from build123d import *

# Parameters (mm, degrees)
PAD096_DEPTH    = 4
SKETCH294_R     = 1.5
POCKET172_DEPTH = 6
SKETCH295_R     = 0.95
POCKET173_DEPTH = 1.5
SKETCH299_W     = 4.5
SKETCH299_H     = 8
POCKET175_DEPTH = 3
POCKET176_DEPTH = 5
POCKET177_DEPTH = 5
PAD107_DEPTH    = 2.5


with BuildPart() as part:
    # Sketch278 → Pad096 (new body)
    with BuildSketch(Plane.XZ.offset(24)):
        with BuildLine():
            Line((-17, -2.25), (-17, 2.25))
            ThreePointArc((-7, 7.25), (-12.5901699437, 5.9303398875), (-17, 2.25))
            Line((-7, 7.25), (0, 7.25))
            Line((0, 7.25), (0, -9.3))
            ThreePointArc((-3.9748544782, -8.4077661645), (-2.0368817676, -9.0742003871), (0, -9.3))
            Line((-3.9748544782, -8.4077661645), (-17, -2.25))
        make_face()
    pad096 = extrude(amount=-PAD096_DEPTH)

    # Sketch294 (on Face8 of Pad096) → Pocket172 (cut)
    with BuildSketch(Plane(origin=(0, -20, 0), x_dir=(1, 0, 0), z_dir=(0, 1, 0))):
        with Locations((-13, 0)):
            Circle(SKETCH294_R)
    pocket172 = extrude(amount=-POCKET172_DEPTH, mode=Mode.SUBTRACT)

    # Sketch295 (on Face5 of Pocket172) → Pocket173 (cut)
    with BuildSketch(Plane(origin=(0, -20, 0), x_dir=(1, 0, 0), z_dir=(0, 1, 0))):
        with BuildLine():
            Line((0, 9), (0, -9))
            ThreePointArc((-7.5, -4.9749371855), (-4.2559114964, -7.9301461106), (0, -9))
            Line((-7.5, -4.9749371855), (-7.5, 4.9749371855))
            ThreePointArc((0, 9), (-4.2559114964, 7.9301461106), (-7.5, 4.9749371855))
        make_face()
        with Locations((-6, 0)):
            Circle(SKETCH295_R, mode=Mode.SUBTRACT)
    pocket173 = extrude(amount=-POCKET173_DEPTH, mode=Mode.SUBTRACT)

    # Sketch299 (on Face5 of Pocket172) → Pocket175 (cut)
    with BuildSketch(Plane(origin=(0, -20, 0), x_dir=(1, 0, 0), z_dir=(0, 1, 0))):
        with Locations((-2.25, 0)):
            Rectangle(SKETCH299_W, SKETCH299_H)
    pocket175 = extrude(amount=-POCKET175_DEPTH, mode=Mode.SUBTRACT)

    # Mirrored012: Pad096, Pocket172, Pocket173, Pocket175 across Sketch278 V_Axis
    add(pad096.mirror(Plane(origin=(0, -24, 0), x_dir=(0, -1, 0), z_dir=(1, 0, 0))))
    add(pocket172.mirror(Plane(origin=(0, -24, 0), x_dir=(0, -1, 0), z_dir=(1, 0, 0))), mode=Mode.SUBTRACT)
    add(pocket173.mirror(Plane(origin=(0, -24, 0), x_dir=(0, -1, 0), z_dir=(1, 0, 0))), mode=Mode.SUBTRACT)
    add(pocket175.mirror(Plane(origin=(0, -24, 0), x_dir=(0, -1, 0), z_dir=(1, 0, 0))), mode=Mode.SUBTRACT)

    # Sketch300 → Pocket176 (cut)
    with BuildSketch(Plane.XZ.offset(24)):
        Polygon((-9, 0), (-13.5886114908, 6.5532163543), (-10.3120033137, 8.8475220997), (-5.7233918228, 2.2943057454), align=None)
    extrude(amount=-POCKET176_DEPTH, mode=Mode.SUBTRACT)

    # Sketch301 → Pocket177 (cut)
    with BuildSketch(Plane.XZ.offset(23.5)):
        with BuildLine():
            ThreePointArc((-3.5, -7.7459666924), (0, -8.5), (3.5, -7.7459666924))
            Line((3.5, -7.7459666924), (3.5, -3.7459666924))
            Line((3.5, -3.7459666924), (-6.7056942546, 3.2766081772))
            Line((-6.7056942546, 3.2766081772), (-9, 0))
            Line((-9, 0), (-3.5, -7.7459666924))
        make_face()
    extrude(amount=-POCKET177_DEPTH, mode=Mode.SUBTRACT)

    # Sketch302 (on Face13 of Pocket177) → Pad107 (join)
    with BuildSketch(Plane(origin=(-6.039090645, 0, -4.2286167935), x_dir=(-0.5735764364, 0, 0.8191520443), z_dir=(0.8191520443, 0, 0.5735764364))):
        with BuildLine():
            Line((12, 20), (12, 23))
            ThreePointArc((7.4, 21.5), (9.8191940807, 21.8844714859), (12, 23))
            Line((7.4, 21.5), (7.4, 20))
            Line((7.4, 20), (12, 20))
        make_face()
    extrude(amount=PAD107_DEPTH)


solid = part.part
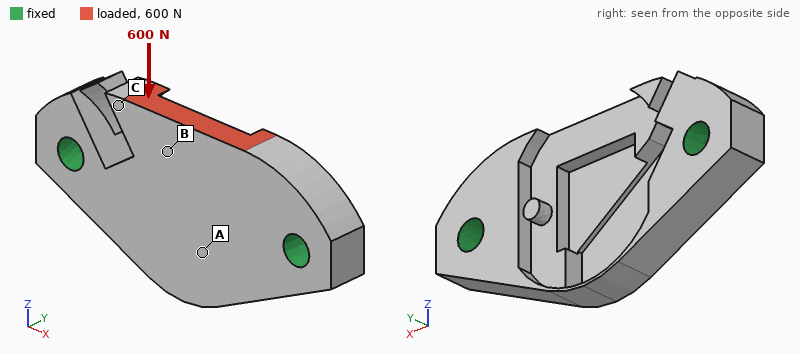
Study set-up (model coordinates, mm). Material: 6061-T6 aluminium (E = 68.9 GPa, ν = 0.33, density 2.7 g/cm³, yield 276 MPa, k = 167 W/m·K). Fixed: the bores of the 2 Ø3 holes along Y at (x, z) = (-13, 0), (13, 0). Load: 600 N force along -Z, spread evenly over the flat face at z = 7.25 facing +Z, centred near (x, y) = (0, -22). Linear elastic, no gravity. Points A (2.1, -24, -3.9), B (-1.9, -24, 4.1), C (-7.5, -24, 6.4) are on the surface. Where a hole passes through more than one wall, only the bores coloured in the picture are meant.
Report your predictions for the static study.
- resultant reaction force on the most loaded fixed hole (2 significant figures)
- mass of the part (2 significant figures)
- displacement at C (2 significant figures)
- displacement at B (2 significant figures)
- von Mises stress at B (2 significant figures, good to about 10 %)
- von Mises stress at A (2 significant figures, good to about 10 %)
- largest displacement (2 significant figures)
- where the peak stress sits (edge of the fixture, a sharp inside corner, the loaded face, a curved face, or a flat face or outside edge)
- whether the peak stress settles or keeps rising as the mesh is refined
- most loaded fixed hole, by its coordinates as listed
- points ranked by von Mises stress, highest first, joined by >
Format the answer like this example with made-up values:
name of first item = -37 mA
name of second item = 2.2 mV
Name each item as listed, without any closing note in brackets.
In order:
resultant reaction force on the most loaded fixed hole = 350 N
mass of the part = 2.7 g
displacement at C = 54 µm
displacement at B = 18 µm
von Mises stress at B = 74 MPa
von Mises stress at A = 44 MPa
largest displacement = 91 µm
where the peak stress sits = a sharp inside corner
whether the peak stress settles or keeps rising as the mesh is refined = keeps rising
most loaded fixed hole, by its coordinates as listed = (13, 0)
points ranked by von Mises stress, highest first, joined by > = B > A > C
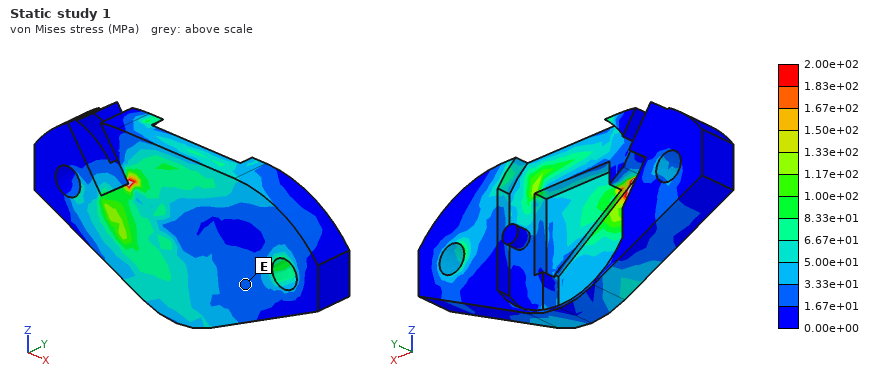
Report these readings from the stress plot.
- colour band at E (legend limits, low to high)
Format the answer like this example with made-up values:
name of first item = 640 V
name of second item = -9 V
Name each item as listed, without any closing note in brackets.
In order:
colour band at E = 1.67e+01 to 3.33e+01 MPa
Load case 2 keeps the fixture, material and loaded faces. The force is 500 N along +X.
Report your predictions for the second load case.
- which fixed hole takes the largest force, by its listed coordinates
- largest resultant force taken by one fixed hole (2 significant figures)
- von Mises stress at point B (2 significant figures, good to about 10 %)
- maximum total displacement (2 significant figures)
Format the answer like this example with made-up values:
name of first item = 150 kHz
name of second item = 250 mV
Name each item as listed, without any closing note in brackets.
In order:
which fixed hole takes the largest force, by its listed coordinates = (13, 0)
largest resultant force taken by one fixed hole = 510 N
von Mises stress at point B = 38 MPa
maximum total displacement = 34 µm
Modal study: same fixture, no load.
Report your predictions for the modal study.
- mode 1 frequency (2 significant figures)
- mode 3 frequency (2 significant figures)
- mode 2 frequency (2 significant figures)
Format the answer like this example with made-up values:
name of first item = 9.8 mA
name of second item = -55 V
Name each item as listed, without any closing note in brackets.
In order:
mode 1 frequency = 9000 Hz
mode 3 frequency = 27 kHz
mode 2 frequency = 25 kHz
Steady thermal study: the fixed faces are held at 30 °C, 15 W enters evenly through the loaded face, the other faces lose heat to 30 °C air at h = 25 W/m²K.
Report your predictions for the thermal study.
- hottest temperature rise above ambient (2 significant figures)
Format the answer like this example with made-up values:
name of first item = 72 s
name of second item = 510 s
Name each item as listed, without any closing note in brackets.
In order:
hottest temperature rise above ambient = 54 K
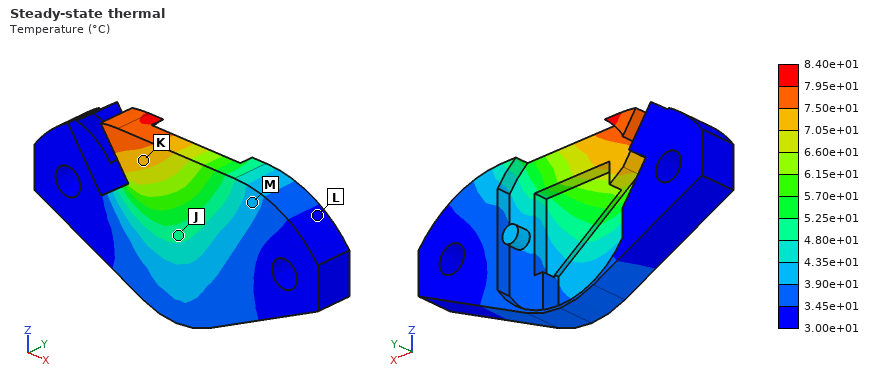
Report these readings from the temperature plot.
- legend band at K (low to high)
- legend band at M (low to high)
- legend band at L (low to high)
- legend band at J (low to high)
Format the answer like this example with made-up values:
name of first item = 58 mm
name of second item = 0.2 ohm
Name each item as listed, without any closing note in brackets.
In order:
legend band at K = 7.05e+01 to 7.50e+01 °C
legend band at M = 3.90e+01 to 4.35e+01 °C
legend band at L = 3.00e+01 to 3.45e+01 °C
legend band at J = 4.80e+01 to 5.25e+01 °C
